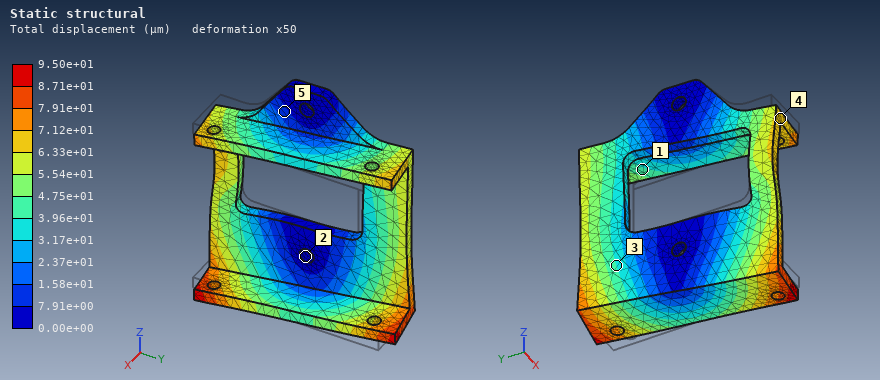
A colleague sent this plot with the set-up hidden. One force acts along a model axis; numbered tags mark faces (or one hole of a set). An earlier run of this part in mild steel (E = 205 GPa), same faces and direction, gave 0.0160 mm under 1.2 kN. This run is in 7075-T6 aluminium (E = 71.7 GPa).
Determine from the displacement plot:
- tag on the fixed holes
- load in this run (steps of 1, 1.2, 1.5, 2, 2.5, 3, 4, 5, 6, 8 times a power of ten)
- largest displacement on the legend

2
2.5 kN
9.50e+01 µm
